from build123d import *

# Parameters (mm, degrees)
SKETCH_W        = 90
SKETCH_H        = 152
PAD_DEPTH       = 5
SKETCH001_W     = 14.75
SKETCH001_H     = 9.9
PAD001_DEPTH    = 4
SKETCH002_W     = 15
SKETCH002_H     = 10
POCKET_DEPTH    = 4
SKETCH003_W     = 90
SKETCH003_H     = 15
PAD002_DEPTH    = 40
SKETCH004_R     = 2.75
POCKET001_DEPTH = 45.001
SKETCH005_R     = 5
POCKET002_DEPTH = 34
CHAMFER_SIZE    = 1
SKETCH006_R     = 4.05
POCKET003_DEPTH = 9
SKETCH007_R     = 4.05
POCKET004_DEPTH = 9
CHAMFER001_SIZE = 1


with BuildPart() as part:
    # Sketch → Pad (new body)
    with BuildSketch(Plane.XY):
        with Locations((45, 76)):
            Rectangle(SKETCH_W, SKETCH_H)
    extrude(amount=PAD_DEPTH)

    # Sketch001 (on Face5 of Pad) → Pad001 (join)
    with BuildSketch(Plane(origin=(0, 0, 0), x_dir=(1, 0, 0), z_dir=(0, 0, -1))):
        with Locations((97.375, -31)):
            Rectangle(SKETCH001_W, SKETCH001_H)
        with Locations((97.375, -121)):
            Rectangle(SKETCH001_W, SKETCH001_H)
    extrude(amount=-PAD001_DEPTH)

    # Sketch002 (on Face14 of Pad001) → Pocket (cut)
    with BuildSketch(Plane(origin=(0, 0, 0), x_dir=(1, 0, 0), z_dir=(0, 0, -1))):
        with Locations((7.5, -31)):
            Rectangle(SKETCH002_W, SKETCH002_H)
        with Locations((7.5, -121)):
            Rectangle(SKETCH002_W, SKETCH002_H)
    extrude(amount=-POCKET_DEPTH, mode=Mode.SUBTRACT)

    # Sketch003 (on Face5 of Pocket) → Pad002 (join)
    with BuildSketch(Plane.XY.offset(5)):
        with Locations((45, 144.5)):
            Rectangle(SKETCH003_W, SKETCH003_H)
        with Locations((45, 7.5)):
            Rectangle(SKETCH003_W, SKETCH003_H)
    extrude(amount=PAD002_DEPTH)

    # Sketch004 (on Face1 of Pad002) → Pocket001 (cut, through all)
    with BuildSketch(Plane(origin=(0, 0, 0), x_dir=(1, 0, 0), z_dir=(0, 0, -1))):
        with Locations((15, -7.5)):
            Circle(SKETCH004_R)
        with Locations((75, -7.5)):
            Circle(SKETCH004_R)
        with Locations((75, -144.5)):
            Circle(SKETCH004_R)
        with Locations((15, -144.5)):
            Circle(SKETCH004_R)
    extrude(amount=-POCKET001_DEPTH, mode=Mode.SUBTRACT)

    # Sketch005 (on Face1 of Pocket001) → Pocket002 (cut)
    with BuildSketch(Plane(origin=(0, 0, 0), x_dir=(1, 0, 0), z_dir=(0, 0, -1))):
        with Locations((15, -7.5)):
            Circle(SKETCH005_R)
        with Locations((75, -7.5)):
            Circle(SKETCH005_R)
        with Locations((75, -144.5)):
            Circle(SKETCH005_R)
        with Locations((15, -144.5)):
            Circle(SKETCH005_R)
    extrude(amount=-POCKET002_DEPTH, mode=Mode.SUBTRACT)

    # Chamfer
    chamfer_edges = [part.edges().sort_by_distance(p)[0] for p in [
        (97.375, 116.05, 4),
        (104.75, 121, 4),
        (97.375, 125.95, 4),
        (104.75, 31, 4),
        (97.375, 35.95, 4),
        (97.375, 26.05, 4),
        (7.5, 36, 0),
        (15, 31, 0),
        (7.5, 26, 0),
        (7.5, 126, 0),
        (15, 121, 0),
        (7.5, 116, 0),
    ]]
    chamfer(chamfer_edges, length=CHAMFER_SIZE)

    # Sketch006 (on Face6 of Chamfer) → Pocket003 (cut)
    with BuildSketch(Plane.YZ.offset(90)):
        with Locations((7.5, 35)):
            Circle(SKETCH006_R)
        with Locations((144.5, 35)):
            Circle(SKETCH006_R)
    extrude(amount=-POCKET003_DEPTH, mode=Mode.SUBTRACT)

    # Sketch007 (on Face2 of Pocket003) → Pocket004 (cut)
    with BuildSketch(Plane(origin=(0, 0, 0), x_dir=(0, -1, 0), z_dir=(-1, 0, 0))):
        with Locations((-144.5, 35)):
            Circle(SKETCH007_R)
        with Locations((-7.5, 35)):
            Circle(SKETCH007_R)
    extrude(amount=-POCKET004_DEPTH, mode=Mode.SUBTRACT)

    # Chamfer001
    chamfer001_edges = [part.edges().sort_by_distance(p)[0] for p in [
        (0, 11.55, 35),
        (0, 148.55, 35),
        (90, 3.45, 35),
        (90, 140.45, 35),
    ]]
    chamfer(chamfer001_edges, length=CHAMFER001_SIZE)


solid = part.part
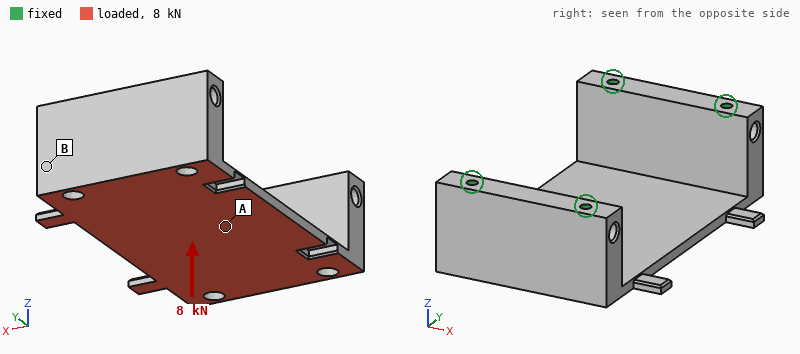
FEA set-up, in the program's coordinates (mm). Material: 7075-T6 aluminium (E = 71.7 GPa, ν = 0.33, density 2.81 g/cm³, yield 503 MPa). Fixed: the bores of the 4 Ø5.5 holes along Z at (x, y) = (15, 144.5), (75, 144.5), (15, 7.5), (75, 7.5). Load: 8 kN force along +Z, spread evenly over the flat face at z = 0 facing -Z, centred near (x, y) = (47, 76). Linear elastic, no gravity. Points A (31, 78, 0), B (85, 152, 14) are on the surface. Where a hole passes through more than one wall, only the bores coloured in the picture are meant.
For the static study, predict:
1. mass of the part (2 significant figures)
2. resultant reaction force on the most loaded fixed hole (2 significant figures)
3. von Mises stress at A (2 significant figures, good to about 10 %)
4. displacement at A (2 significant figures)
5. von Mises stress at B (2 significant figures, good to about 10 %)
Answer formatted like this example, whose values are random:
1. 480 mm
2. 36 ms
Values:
1. 460 g
2. 2.6 kN
3. 97 MPa
4. 0.57 mm
5. 17 MPa
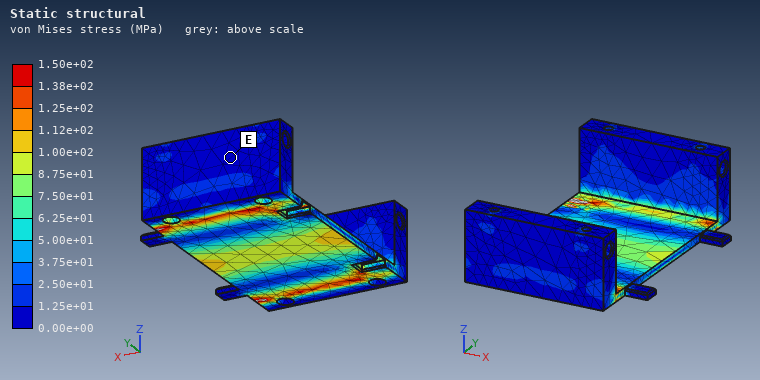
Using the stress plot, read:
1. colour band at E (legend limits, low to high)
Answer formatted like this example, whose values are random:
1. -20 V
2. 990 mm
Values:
1. 0.00e+00 to 1.25e+01 MPa
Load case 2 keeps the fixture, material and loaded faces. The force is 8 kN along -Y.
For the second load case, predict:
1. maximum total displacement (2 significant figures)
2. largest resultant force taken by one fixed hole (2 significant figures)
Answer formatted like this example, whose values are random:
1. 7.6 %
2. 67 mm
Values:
1. 0.14 mm
2. 2.0 kN
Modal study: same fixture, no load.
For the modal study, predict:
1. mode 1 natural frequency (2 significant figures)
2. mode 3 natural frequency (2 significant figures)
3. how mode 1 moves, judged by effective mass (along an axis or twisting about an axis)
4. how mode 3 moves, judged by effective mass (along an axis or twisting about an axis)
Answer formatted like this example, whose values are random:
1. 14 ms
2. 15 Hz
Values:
1. 1500 Hz
2. 2500 Hz
3. along Z
4. along Y
